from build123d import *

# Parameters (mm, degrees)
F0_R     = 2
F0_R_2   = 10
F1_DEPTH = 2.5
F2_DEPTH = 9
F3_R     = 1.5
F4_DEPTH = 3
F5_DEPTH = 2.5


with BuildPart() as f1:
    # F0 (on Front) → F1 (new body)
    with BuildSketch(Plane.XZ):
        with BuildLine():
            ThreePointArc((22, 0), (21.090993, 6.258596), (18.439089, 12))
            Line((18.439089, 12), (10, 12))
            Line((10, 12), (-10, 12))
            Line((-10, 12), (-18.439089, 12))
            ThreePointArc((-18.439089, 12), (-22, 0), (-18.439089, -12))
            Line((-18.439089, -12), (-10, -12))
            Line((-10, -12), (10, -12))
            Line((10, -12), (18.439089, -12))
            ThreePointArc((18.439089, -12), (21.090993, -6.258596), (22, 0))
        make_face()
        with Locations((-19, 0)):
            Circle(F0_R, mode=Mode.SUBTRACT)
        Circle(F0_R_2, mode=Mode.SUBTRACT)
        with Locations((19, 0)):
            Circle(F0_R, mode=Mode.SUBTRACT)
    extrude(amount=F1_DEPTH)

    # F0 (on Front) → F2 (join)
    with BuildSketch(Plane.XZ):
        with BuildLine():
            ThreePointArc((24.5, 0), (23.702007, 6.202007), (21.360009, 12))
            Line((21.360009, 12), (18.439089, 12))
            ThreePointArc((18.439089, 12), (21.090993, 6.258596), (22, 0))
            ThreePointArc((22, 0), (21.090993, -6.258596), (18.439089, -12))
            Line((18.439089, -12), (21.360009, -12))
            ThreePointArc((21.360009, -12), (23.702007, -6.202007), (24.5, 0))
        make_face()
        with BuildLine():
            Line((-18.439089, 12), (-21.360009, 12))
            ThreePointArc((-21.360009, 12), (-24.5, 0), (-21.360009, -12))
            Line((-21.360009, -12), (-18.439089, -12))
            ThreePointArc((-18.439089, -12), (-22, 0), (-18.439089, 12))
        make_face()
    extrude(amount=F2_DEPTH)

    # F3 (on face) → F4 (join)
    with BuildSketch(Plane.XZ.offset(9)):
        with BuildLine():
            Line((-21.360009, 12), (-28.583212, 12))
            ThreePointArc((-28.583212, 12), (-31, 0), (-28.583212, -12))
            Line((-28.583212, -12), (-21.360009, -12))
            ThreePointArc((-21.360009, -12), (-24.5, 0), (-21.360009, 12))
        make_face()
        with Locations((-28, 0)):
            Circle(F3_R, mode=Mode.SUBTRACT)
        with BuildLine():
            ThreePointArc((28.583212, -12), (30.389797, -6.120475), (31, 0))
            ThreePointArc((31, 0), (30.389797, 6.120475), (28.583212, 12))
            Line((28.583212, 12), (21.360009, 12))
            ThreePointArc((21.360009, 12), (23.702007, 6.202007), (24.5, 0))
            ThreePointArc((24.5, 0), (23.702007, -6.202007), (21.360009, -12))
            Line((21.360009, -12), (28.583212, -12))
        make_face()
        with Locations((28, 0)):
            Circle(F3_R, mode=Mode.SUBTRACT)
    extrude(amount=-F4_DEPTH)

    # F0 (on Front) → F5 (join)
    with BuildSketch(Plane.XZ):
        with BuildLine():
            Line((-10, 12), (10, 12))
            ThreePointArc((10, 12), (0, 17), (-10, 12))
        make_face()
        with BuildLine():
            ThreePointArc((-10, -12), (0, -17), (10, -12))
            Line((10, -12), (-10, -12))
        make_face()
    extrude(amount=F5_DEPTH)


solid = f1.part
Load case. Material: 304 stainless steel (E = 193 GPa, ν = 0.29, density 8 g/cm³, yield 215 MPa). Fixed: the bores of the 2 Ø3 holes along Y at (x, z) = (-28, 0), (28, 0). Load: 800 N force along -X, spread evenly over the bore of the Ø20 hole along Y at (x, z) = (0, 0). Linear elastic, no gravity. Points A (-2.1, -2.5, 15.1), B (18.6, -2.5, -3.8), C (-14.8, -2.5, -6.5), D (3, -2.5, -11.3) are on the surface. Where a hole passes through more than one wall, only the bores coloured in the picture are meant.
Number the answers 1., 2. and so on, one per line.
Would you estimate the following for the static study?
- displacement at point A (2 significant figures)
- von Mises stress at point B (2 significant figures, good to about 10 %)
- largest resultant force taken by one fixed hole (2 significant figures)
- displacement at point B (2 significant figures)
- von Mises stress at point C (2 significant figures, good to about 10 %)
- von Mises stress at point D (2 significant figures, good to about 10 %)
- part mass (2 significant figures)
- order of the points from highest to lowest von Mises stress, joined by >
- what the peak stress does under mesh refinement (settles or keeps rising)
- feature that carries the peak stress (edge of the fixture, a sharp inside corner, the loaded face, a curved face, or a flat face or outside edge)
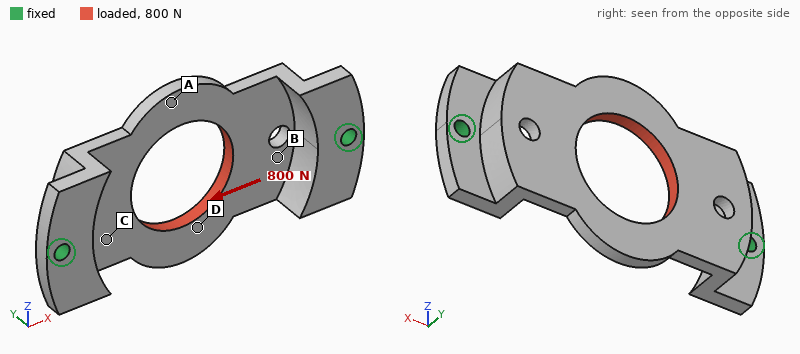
1. 10 µm
2. 42 MPa
3. 400 N
4. 10 µm
5. 34 MPa
6. 18 MPa
7. 33 g
8. B > C > D > A
9. keeps rising
10. edge of the fixture
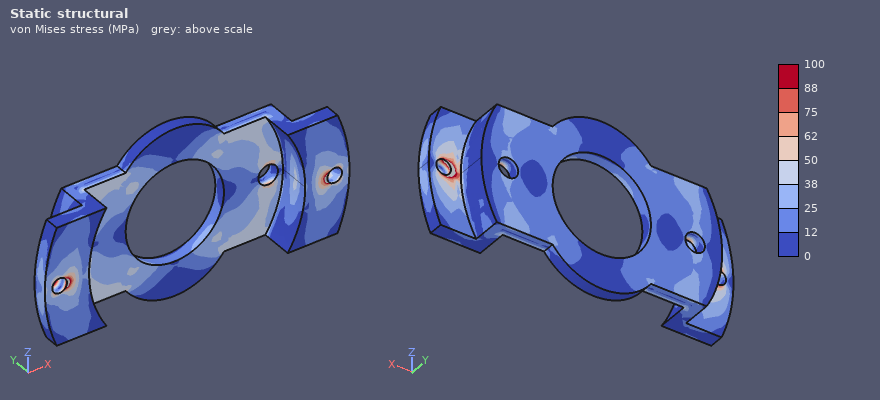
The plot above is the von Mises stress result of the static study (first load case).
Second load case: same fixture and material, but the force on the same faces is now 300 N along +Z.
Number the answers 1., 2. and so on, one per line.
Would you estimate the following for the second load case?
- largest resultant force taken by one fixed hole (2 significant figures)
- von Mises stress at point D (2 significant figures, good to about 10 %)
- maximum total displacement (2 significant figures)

1. 150 N
2. 8.0 MPa
3. 10 µm
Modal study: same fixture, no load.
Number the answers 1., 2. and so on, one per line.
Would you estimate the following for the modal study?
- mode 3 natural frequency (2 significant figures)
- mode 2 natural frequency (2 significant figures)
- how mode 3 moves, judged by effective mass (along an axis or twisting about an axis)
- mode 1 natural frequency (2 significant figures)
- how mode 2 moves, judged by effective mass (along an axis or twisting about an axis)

1. 7500 Hz
2. 5500 Hz
3. along X
4. 4900 Hz
5. along Y
